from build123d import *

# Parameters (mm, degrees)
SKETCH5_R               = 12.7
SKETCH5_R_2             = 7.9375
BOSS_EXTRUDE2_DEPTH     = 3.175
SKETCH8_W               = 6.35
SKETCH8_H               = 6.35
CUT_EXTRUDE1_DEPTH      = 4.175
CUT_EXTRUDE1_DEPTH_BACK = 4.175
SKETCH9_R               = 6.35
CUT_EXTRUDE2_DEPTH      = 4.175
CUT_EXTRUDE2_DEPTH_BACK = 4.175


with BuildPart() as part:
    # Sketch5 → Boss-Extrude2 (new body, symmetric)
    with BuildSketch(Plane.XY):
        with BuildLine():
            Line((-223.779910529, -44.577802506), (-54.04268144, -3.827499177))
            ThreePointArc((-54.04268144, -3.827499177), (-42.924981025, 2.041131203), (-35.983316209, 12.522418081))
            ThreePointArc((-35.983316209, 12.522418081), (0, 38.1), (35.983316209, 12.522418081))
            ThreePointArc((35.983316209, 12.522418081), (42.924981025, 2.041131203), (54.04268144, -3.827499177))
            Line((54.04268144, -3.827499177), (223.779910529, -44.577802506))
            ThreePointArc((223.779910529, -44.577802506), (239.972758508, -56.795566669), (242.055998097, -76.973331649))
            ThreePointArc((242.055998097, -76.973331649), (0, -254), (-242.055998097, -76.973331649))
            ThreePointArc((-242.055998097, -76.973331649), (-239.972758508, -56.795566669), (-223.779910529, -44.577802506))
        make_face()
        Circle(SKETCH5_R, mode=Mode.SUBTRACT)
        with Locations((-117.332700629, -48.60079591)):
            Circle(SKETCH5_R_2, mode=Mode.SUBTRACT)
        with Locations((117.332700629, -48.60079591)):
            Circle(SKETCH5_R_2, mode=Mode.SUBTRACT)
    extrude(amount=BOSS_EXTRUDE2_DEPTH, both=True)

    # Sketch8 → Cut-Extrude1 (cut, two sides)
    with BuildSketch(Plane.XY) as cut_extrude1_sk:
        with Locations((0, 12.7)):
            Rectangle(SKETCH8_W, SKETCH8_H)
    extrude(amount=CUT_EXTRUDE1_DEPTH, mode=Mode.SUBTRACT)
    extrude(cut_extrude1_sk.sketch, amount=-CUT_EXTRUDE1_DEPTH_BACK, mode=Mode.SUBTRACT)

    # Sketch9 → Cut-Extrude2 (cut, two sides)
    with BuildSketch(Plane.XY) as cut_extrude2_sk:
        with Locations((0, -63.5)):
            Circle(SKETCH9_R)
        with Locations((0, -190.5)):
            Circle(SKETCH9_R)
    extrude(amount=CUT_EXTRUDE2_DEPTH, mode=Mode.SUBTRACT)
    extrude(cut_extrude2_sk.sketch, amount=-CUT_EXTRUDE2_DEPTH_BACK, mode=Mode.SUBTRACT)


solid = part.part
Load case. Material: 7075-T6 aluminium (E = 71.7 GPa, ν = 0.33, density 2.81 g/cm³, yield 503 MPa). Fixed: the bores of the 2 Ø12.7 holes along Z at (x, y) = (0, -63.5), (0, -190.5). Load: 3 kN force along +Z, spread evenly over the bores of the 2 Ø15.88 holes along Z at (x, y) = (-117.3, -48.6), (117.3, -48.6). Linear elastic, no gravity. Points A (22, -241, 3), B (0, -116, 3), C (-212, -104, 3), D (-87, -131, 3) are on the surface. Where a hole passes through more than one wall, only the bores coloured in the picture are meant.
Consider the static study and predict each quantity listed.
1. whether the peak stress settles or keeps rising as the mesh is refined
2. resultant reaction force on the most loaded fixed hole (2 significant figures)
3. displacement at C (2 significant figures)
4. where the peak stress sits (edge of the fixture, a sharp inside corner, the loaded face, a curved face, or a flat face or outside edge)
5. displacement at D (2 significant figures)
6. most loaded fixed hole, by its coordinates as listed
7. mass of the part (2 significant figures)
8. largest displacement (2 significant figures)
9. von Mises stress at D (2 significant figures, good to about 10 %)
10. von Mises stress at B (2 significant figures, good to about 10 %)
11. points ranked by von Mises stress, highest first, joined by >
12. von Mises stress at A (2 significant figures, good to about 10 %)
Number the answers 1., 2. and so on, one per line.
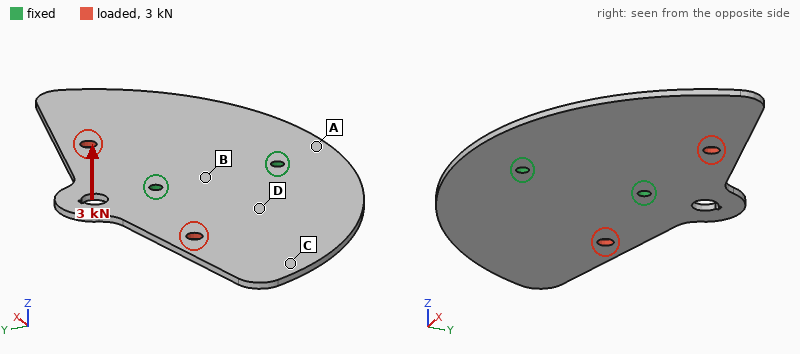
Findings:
1. keeps rising
2. 3.0 kN
3. 4.5 mm
4. edge of the fixture
5. 1.1 mm
6. (0, -63.5)
7. 1.6 kg
8. 6.0 mm
9. 44 MPa
10. 83 MPa
11. B > D > A > C
12. 28 MPa
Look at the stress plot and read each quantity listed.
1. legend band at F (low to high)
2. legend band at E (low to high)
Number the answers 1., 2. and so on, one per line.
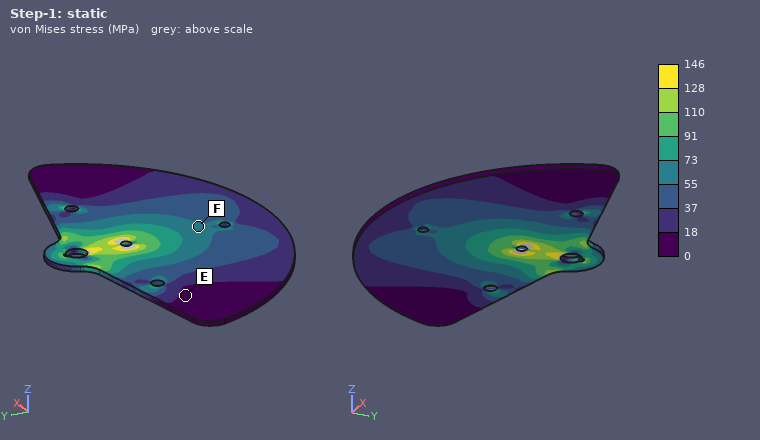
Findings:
1. 55 to 73 MPa
2. 0 to 18 MPa
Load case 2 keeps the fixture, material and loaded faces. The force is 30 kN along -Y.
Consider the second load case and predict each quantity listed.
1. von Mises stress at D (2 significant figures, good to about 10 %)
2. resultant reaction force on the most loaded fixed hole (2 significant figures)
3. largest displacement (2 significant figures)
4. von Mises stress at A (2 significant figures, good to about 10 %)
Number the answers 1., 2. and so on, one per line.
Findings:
1. 21 MPa
2. 15 kN
3. 0.10 mm
4. 22 MPa
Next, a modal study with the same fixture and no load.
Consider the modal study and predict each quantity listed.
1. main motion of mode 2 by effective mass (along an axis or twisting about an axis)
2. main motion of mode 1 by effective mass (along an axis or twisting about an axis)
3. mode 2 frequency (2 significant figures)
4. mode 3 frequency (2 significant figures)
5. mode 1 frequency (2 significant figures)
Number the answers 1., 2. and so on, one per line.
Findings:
1. along Z
2. twisting about Y
3. 130 Hz
4. 360 Hz
5. 120 Hz
